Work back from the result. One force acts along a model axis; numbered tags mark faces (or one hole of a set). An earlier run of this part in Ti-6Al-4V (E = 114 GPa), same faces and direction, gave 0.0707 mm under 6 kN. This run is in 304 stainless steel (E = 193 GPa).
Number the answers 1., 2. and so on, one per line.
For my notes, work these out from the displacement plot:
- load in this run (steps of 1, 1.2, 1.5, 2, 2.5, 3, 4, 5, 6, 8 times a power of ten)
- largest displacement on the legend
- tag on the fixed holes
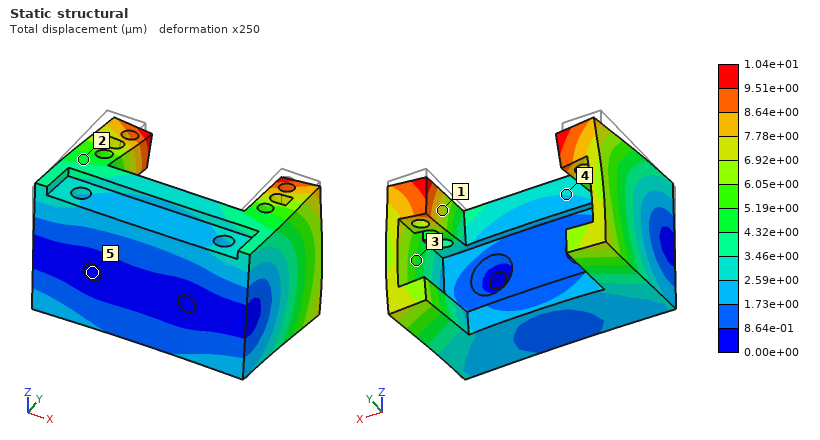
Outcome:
1. 1.5 kN
2. 1.04e+01 µm
3. 5
